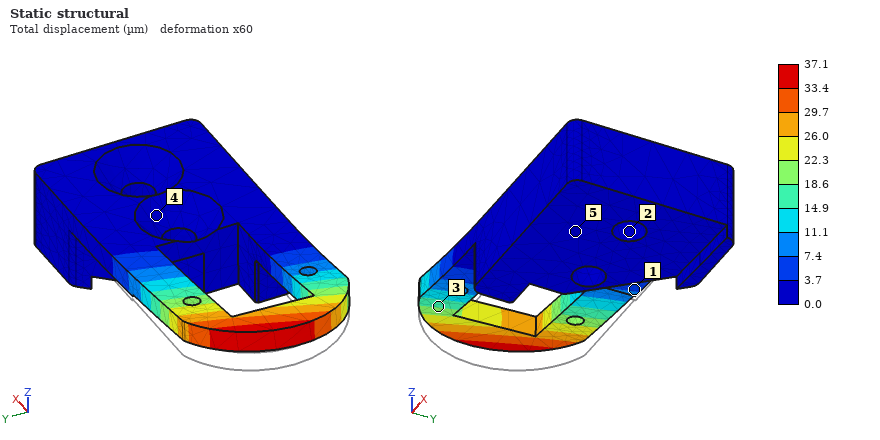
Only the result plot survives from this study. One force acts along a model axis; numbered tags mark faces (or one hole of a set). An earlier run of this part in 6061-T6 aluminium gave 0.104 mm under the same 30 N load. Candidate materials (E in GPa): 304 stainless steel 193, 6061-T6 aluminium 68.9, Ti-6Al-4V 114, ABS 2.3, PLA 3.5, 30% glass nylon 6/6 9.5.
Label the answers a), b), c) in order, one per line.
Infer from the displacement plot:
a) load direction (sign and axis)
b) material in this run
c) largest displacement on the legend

a) +Z
b) 304 stainless steel
c) 37.1 µm
